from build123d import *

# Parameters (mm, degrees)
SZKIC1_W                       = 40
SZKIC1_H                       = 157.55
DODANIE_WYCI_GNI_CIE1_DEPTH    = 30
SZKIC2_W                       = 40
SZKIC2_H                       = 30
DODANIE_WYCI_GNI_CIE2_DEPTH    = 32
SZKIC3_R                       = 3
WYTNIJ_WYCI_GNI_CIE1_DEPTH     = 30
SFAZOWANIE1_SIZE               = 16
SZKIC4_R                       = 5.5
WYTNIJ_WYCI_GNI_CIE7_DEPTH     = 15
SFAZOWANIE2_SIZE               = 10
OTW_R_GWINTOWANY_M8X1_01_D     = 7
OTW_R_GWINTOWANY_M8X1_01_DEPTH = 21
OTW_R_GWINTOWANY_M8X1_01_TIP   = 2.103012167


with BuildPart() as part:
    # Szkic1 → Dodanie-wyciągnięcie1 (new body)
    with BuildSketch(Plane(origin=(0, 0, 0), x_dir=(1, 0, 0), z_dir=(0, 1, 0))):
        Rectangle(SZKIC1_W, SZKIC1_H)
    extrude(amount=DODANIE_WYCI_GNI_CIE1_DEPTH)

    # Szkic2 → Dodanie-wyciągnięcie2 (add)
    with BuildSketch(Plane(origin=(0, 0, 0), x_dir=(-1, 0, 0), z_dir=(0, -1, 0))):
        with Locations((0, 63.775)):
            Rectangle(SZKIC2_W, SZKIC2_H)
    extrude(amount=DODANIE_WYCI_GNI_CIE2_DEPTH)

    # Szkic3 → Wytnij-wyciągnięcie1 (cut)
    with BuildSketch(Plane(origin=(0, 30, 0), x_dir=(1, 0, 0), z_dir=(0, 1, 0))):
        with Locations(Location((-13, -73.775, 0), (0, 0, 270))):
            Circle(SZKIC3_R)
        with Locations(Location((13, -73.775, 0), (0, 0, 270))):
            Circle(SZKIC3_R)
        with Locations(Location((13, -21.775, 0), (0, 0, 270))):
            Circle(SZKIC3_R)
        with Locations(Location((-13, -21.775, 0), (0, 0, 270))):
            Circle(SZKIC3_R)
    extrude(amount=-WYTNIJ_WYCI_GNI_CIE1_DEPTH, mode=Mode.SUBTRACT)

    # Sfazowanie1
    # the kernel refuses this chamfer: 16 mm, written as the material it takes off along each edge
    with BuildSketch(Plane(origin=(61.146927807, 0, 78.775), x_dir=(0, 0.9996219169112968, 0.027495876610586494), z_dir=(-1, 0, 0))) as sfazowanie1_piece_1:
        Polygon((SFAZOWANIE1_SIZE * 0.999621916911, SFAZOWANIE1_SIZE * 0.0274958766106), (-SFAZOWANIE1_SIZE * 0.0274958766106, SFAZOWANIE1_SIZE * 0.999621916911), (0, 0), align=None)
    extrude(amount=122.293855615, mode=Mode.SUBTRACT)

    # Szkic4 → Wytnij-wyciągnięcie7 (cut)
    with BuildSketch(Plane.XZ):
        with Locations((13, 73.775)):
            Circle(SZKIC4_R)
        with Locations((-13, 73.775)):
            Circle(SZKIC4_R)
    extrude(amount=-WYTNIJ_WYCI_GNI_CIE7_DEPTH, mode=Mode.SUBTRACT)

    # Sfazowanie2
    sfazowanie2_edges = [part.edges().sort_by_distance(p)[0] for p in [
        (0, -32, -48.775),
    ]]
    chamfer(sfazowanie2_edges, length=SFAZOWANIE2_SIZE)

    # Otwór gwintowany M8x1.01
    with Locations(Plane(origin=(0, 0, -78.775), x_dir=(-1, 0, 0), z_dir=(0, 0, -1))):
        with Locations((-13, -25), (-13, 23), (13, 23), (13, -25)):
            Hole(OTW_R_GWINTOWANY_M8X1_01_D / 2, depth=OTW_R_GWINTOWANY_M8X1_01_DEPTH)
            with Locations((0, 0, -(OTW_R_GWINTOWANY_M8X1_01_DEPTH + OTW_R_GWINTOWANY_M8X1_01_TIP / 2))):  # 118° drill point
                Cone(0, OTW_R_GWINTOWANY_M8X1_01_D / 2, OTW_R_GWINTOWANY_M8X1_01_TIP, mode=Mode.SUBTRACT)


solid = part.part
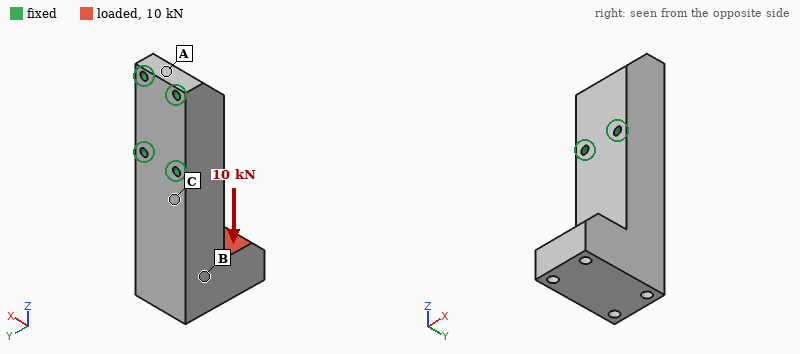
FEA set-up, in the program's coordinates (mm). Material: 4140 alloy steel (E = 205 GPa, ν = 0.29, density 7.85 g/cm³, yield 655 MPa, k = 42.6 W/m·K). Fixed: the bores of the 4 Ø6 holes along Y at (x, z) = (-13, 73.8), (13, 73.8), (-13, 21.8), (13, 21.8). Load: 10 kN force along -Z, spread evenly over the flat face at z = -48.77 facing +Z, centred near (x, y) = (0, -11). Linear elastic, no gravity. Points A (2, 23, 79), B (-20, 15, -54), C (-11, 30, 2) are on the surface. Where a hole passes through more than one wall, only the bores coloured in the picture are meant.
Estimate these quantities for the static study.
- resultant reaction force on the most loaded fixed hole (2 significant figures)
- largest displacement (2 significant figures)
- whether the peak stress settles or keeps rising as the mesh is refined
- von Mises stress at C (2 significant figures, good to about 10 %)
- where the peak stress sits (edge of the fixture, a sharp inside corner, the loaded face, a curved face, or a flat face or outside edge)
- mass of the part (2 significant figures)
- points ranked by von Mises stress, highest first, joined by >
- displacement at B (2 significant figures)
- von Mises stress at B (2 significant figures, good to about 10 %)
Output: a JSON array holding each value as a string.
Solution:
["4.8 kN", "94 µm", "keeps rising", "35 MPa", "edge of the fixture", "1.7 kg", "C > B > A", "41 µm", "17 MPa"]
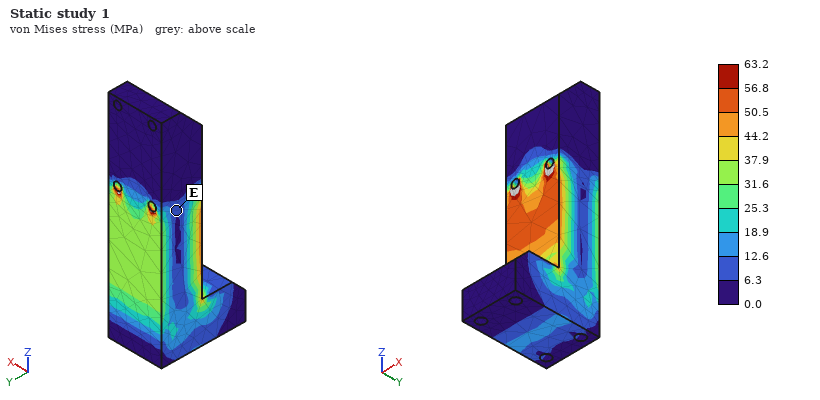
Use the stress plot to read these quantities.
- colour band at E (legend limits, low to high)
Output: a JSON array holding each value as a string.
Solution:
["6.3 to 12.6 MPa"]
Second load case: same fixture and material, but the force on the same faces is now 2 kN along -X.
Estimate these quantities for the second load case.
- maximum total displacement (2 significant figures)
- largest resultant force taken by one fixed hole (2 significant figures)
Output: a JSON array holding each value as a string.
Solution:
["25 µm", "4.9 kN"]
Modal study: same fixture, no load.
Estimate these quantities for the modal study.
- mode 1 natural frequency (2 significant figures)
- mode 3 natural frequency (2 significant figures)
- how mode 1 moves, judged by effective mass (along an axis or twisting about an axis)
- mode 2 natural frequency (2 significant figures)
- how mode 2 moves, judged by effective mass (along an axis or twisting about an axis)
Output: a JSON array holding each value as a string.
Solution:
["1700 Hz", "4500 Hz", "along Y", "2100 Hz", "along X"]
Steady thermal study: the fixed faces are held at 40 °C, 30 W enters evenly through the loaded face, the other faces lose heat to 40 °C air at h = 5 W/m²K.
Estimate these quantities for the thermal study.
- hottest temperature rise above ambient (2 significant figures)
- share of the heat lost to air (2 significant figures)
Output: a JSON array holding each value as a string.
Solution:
["57 K", "11 %"]
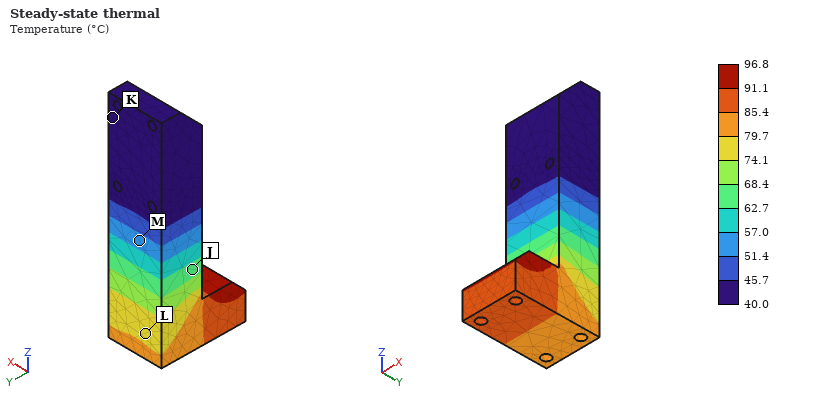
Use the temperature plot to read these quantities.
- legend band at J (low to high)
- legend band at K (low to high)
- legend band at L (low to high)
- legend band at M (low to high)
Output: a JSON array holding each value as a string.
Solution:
["62.7 to 68.4 °C", "40.0 to 45.7 °C", "74.1 to 79.7 °C", "51.4 to 57.0 °C"]
